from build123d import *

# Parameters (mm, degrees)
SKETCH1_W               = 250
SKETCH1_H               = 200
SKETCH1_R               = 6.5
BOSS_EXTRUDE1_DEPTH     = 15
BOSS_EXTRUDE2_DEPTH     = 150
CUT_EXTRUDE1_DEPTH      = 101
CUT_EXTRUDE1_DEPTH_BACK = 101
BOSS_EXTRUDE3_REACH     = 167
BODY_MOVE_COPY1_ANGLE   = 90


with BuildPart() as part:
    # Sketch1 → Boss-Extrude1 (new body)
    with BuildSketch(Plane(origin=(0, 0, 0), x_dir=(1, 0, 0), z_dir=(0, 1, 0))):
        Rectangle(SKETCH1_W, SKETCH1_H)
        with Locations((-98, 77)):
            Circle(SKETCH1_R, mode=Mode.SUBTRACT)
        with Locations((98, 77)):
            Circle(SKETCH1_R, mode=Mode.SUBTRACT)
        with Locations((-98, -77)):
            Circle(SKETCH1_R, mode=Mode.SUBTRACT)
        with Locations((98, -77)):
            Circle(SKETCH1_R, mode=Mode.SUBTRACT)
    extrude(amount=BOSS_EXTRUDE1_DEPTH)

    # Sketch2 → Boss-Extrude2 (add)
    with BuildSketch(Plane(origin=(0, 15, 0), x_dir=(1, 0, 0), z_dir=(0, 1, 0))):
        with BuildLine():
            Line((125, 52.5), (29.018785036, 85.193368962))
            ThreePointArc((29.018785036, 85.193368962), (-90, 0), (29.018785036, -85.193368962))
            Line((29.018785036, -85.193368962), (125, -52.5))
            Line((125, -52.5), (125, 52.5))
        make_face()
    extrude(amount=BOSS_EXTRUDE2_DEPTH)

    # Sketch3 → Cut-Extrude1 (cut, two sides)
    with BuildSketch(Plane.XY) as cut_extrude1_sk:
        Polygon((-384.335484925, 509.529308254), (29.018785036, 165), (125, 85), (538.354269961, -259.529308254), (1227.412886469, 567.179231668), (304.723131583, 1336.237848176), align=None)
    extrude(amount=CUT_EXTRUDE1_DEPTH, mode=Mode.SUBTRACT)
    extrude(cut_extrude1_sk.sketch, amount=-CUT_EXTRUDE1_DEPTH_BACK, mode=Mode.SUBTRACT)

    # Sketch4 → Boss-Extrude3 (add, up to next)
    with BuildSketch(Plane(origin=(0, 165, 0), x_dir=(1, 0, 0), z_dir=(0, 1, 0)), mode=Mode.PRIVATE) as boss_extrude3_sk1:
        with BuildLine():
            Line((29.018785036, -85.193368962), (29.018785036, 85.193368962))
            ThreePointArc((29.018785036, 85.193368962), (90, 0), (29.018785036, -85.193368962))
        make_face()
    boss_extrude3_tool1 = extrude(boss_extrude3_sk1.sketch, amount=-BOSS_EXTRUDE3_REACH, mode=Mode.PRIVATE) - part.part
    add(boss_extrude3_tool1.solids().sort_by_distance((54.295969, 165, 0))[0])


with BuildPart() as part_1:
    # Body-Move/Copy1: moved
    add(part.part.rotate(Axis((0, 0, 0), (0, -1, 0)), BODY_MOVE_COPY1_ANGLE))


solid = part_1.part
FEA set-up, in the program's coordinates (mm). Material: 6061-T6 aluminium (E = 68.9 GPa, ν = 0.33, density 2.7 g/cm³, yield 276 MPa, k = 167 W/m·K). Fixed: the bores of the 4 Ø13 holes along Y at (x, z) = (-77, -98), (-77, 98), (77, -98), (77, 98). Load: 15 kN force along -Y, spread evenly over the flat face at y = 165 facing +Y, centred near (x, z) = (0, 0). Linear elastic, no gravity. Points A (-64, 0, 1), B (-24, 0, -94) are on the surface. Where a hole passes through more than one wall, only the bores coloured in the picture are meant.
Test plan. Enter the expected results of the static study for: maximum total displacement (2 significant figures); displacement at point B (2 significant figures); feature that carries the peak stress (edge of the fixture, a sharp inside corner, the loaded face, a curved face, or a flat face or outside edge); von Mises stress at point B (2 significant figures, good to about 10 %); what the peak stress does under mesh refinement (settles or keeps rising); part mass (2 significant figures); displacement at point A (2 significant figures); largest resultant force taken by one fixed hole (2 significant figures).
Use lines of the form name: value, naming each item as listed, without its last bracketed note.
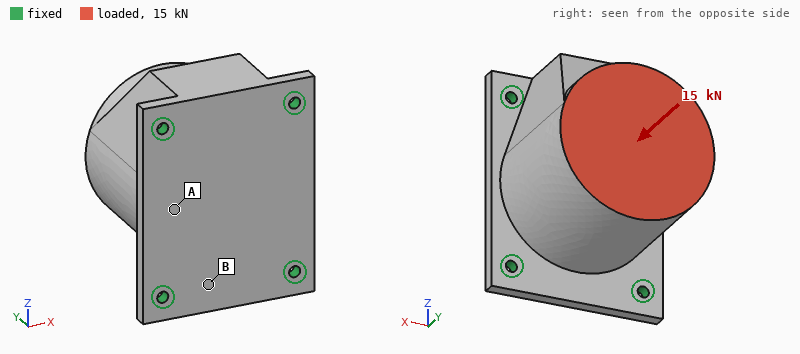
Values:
maximum total displacement: 35 µm
displacement at point B: 25 µm
feature that carries the peak stress: edge of the fixture
von Mises stress at point B: 8.8 MPa
what the peak stress does under mesh refinement: keeps rising
part mass: 14 kg
displacement at point A: 19 µm
largest resultant force taken by one fixed hole: 4.1 kN
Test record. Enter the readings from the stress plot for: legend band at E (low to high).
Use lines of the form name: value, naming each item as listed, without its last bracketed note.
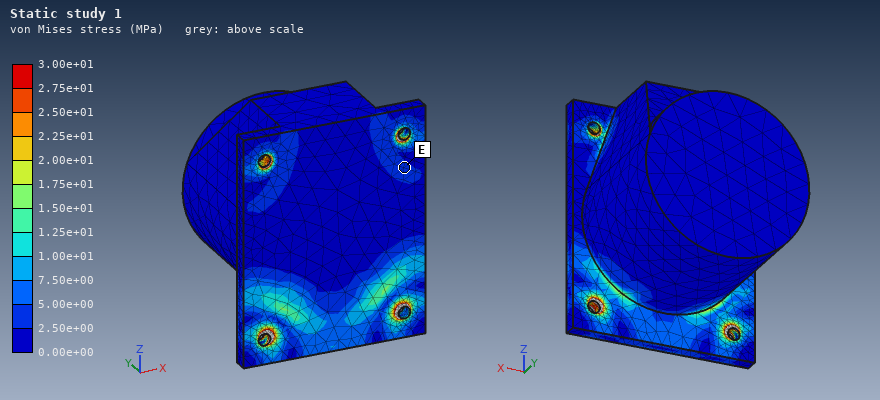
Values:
legend band at E: 2.50e+00 to 5.00e+00 MPa
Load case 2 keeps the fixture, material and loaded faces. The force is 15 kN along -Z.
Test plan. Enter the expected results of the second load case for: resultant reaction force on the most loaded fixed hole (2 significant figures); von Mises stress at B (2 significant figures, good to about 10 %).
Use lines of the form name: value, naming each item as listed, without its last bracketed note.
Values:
resultant reaction force on the most loaded fixed hole: 7.9 kN
von Mises stress at B: 15 MPa
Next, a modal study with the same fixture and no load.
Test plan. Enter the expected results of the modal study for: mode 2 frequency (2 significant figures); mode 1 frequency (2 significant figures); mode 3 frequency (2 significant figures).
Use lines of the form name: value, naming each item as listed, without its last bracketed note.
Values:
mode 2 frequency: 1000 Hz
mode 1 frequency: 990 Hz
mode 3 frequency: 1600 Hz
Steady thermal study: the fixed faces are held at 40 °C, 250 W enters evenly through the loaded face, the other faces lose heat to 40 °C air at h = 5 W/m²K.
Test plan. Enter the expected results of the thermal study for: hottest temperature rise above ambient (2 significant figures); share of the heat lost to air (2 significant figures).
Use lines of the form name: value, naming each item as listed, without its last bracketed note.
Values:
hottest temperature rise above ambient: 21 K
share of the heat lost to air: 4.7 %
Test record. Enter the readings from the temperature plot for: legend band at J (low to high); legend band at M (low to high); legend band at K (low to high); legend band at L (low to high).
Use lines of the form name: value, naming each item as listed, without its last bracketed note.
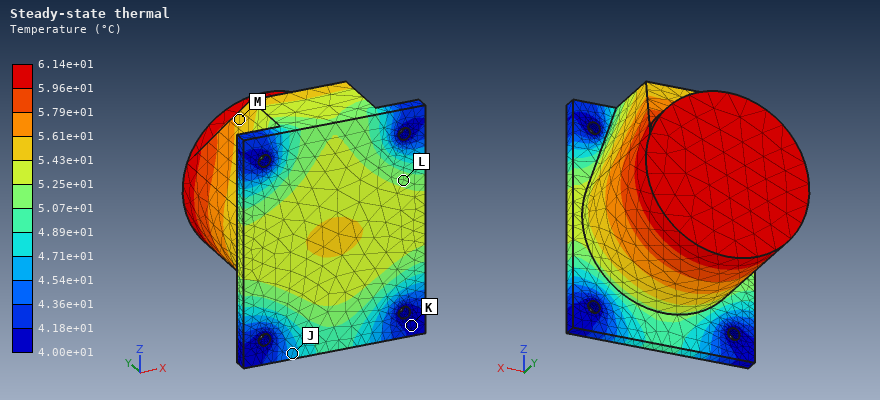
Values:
legend band at J: 4.54e+01 to 4.71e+01 °C
legend band at M: 5.43e+01 to 5.61e+01 °C
legend band at K: 4.00e+01 to 4.18e+01 °C
legend band at L: 5.07e+01 to 5.25e+01 °C
